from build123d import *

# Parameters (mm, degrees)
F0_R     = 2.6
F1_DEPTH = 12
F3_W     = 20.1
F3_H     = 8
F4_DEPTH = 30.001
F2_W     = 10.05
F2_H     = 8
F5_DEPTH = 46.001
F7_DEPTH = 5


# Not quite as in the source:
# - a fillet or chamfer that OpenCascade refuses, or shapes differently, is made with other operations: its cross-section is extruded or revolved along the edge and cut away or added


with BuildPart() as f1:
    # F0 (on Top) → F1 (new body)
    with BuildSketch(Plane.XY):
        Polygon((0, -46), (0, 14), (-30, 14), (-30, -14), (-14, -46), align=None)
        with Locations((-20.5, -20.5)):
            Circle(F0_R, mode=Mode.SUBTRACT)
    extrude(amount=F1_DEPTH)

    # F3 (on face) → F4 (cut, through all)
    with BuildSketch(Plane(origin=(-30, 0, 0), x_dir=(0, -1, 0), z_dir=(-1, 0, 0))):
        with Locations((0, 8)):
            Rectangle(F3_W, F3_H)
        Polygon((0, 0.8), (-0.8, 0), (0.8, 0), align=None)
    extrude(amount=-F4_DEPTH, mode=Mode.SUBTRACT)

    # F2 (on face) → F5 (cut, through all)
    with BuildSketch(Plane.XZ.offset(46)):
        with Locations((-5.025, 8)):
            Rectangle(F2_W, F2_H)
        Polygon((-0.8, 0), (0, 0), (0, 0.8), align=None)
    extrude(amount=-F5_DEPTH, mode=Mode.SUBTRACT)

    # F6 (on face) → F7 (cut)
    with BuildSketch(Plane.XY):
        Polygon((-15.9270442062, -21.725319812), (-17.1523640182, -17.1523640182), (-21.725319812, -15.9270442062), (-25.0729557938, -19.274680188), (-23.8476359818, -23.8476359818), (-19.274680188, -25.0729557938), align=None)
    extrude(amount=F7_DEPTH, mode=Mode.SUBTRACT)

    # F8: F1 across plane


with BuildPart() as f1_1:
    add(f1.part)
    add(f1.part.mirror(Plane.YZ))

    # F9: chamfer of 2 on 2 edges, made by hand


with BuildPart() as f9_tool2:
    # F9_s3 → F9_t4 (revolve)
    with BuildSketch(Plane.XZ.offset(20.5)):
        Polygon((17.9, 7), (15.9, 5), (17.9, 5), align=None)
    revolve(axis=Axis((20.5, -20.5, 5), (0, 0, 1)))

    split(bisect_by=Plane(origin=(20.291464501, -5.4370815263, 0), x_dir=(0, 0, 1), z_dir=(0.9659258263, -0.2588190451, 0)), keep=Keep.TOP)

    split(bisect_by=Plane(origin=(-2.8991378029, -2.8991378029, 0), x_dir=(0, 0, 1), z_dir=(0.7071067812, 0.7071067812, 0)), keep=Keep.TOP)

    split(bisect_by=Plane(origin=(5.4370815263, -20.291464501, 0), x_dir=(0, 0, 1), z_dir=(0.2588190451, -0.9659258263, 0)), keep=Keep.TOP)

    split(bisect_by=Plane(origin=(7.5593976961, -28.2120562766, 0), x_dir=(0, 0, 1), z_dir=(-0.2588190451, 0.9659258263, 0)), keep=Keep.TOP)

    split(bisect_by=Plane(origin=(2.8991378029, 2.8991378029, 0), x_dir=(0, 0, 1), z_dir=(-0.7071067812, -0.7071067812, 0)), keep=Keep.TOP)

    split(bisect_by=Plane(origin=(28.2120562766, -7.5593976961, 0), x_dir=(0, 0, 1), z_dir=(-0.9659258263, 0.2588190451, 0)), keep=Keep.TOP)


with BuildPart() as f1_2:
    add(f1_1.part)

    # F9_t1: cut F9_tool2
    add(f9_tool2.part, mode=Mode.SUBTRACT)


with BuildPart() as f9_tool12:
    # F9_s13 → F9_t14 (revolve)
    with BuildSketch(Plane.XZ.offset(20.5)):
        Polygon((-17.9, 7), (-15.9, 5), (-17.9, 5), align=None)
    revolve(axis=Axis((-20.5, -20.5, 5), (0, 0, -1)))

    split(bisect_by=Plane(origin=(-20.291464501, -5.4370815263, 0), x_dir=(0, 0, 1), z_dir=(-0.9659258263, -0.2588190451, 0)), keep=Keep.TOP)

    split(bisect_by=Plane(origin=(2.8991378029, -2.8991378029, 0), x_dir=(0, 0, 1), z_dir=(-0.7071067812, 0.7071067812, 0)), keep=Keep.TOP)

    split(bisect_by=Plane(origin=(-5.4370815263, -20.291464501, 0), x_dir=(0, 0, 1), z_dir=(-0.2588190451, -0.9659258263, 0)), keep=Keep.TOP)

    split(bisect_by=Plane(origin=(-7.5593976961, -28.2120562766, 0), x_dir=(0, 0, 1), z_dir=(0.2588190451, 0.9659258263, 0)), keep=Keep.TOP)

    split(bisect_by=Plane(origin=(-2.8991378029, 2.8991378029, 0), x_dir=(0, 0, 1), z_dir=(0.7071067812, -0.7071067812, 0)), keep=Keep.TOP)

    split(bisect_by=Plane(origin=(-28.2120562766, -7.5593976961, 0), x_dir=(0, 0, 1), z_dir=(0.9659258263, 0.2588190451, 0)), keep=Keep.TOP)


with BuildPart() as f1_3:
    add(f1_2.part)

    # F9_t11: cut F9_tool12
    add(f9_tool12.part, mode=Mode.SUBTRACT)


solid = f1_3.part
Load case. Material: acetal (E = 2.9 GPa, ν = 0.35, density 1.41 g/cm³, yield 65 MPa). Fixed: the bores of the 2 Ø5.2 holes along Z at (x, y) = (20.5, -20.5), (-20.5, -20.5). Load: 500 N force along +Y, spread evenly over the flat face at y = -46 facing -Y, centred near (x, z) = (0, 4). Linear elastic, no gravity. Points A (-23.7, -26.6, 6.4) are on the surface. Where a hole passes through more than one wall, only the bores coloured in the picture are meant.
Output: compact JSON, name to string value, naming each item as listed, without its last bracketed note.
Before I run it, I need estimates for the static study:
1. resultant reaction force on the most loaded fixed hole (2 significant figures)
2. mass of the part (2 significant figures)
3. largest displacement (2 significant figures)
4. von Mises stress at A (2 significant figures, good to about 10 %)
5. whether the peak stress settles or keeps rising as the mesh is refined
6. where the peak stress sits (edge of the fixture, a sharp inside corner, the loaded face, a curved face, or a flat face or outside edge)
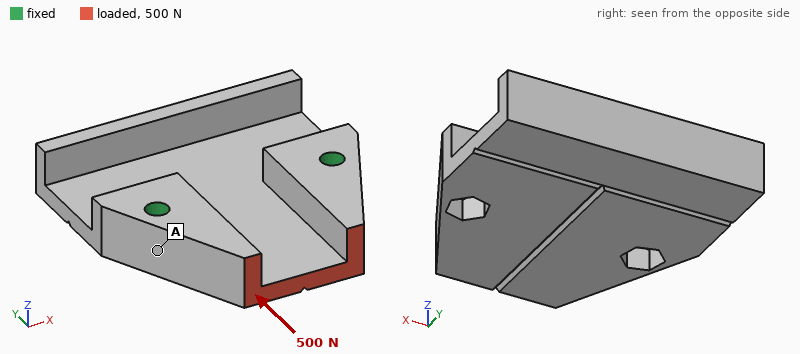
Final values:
{"resultant reaction force on the most loaded fixed hole": "250 N", "mass of the part": "29 g", "largest displacement": "0.15 mm", "von Mises stress at A": "2.5 MPa", "whether the peak stress settles or keeps rising as the mesh is refined": "keeps rising", "where the peak stress sits": "edge of the fixture"}
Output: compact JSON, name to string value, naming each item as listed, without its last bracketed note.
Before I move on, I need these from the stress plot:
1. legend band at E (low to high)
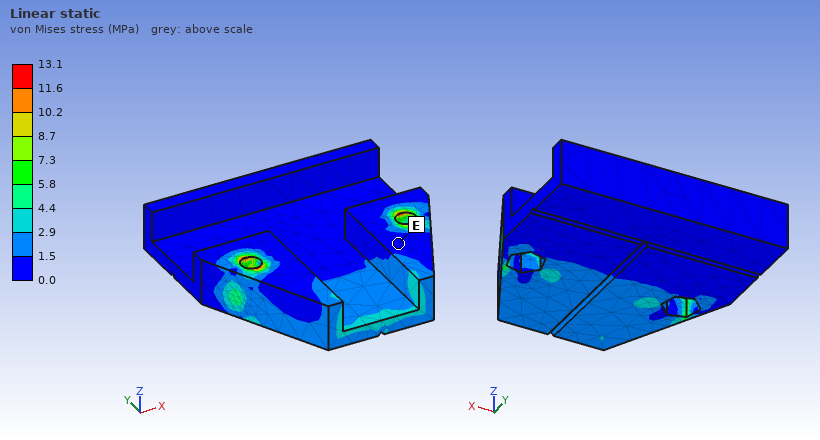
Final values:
{"legend band at E": "0.0 to 1.5 MPa"}
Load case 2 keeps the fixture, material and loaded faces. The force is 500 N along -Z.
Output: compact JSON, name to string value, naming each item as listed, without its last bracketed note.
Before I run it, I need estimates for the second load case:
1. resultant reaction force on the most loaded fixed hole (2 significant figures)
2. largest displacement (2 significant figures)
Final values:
{"resultant reaction force on the most loaded fixed hole": "350 N", "largest displacement": "0.99 mm"}
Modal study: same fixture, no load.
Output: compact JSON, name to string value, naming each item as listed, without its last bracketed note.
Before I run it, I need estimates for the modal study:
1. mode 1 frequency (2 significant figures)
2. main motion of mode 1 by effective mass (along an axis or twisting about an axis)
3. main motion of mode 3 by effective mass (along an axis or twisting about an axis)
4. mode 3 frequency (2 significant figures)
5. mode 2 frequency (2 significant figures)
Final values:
{"mode 1 frequency": "770 Hz", "main motion of mode 1 by effective mass": "along Z", "main motion of mode 3 by effective mass": "along Y", "mode 3 frequency": "2200 Hz", "mode 2 frequency": "1300 Hz"}
